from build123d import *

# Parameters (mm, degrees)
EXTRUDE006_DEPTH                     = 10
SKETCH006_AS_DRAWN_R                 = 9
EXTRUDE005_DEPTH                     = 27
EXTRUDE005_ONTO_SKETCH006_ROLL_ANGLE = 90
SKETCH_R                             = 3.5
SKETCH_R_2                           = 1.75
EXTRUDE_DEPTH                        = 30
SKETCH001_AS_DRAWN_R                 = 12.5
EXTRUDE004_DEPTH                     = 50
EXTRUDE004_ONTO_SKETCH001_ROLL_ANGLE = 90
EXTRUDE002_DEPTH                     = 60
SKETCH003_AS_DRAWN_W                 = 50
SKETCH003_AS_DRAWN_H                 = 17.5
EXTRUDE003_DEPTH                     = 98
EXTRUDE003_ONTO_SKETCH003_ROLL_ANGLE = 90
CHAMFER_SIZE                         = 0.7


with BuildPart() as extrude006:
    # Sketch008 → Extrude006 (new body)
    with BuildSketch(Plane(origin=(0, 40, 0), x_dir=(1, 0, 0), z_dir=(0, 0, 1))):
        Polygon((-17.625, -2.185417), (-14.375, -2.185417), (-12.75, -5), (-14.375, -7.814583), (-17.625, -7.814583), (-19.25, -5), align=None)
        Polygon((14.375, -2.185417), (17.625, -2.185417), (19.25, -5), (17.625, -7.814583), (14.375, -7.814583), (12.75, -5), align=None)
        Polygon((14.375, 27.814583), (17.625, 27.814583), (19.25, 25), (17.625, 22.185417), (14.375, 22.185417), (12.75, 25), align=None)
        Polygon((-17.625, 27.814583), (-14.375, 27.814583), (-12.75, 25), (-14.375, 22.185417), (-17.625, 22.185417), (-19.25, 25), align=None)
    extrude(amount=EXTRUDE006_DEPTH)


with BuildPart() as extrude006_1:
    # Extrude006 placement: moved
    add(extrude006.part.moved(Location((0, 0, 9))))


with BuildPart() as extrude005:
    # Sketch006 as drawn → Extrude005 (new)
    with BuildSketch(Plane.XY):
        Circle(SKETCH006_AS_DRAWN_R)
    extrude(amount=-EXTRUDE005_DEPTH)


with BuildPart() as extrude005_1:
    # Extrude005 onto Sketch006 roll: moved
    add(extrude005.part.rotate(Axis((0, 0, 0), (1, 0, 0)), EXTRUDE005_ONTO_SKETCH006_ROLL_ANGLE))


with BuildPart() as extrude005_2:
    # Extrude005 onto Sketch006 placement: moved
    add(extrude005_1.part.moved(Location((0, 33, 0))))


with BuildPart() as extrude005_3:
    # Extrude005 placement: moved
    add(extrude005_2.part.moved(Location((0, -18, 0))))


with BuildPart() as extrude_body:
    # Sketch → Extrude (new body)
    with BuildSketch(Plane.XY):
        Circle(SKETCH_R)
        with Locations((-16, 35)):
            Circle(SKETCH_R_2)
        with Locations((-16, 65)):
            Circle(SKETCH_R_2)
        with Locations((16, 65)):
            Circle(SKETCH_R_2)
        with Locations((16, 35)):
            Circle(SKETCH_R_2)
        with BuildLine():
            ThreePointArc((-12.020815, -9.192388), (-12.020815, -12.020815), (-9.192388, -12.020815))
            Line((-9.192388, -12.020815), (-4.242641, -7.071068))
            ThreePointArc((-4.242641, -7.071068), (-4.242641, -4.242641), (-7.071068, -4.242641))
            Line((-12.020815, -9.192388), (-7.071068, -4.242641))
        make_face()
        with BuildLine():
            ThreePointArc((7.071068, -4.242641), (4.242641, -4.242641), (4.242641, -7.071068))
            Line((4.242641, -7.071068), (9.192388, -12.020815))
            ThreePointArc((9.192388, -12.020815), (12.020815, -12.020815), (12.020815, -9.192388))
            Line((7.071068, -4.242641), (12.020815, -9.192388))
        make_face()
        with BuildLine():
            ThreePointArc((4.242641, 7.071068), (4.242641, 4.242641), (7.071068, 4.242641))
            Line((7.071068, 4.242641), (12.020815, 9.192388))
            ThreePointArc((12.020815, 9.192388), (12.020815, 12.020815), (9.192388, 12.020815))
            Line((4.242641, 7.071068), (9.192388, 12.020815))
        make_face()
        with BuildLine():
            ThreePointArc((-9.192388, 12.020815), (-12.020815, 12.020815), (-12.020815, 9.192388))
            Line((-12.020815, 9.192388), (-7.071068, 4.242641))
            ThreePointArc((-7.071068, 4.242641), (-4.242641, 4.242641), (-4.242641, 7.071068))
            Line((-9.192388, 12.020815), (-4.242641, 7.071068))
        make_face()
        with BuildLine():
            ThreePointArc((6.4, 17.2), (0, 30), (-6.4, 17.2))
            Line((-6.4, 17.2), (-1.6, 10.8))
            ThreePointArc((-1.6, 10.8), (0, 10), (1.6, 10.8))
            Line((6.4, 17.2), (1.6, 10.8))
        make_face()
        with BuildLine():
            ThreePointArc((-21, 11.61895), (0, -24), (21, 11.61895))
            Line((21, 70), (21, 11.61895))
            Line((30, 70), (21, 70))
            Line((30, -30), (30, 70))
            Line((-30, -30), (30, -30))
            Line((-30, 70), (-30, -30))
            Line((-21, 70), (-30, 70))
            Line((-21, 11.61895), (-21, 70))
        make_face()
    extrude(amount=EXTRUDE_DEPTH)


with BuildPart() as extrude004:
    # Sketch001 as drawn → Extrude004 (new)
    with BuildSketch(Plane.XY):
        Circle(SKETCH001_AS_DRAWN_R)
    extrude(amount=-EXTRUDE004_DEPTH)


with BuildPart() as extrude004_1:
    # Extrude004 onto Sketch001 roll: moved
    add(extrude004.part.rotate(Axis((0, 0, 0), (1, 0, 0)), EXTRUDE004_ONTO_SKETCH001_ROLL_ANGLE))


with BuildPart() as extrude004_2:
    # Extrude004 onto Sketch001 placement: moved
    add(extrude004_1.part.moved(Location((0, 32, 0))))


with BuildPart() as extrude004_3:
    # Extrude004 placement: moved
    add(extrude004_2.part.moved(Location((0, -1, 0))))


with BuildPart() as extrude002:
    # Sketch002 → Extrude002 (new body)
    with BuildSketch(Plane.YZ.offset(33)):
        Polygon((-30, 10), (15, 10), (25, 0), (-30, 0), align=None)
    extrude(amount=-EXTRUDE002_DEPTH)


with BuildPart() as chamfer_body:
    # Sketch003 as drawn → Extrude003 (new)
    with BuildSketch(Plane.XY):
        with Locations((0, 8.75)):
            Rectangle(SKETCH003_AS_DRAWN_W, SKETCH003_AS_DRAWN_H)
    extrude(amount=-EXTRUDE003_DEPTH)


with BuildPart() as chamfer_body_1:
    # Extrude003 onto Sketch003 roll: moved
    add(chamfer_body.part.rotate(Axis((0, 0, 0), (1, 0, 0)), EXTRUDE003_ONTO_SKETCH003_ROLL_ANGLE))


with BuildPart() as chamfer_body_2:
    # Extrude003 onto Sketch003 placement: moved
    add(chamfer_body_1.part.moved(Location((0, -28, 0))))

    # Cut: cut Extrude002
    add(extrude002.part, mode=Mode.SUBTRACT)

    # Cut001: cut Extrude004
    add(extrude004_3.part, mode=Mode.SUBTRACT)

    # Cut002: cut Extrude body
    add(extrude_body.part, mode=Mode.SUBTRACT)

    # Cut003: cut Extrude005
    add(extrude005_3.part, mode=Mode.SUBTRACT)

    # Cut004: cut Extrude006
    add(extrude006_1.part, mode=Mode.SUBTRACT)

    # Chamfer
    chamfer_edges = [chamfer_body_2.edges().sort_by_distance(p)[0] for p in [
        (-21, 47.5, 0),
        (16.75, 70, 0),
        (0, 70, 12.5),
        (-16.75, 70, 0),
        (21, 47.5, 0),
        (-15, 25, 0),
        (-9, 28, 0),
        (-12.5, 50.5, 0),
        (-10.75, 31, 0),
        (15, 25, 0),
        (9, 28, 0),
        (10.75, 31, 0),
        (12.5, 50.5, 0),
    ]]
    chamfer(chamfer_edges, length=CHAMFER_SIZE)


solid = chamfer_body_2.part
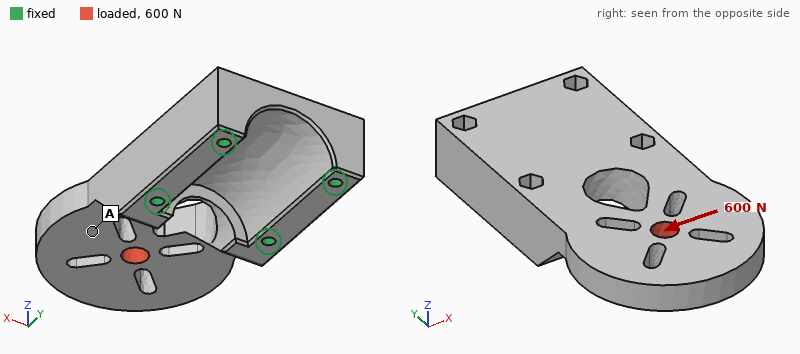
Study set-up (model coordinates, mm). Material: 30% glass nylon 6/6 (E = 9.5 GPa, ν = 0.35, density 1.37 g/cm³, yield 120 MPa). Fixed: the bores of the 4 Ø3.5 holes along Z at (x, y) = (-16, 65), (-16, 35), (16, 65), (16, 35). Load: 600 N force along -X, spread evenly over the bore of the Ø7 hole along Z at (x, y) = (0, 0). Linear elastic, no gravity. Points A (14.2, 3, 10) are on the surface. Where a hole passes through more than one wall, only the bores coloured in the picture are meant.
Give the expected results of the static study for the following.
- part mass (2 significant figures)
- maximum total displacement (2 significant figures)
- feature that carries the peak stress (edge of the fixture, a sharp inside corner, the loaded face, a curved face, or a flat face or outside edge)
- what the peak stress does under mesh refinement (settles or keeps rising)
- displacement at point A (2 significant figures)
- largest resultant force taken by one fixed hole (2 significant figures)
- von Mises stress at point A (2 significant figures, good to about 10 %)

47 g
0.11 mm
edge of the fixture
keeps rising
0.078 mm
530 N
3.2 MPa
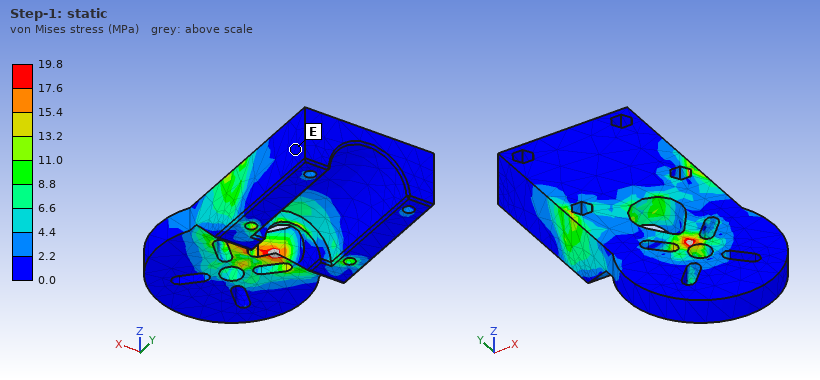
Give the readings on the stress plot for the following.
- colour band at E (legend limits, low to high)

0.0 to 2.2 MPa
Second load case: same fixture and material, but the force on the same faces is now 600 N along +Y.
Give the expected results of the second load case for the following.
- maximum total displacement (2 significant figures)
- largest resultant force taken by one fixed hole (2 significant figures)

64 µm
200 N
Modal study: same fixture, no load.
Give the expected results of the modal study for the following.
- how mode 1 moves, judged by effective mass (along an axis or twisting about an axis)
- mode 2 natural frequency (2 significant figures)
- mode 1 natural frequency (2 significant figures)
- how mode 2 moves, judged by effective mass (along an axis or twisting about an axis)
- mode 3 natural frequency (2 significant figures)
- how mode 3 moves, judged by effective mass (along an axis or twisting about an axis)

along Z
3000 Hz
1300 Hz
along X
3700 Hz
along X
